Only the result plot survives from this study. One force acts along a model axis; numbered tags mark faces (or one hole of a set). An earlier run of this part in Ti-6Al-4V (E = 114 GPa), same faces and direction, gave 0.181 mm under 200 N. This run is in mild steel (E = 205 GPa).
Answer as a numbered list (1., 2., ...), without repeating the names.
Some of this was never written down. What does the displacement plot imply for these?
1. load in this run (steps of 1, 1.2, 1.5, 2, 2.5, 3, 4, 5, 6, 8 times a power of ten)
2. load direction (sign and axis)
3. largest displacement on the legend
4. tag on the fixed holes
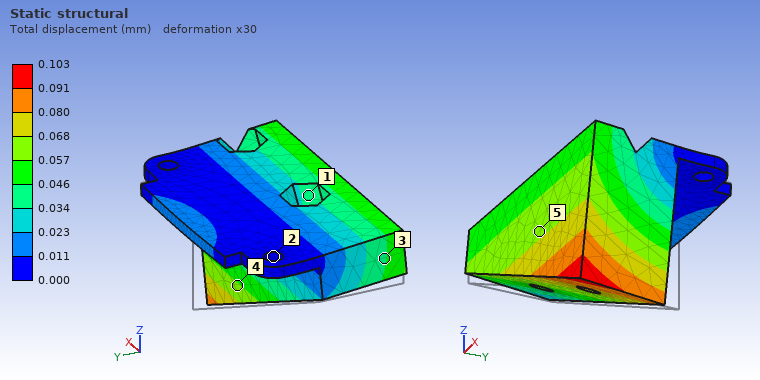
1. 200 N
2. -Y
3. 0.103 mm
4. 2
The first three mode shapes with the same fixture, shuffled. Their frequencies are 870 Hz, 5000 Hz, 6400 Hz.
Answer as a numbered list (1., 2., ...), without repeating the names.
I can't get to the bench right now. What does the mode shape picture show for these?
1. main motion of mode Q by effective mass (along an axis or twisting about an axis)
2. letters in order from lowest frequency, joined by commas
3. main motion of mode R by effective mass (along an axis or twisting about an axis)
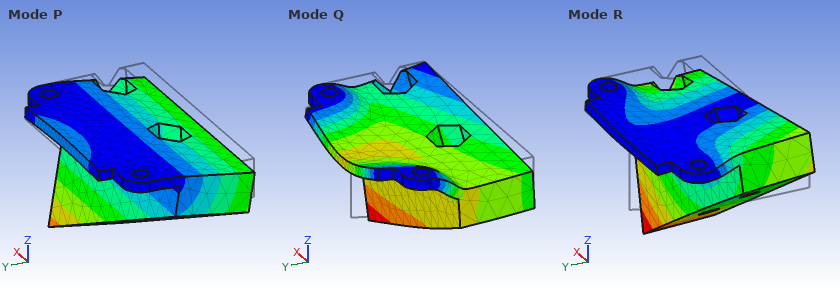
1. along Z
2. P, R, Q
3. along X
